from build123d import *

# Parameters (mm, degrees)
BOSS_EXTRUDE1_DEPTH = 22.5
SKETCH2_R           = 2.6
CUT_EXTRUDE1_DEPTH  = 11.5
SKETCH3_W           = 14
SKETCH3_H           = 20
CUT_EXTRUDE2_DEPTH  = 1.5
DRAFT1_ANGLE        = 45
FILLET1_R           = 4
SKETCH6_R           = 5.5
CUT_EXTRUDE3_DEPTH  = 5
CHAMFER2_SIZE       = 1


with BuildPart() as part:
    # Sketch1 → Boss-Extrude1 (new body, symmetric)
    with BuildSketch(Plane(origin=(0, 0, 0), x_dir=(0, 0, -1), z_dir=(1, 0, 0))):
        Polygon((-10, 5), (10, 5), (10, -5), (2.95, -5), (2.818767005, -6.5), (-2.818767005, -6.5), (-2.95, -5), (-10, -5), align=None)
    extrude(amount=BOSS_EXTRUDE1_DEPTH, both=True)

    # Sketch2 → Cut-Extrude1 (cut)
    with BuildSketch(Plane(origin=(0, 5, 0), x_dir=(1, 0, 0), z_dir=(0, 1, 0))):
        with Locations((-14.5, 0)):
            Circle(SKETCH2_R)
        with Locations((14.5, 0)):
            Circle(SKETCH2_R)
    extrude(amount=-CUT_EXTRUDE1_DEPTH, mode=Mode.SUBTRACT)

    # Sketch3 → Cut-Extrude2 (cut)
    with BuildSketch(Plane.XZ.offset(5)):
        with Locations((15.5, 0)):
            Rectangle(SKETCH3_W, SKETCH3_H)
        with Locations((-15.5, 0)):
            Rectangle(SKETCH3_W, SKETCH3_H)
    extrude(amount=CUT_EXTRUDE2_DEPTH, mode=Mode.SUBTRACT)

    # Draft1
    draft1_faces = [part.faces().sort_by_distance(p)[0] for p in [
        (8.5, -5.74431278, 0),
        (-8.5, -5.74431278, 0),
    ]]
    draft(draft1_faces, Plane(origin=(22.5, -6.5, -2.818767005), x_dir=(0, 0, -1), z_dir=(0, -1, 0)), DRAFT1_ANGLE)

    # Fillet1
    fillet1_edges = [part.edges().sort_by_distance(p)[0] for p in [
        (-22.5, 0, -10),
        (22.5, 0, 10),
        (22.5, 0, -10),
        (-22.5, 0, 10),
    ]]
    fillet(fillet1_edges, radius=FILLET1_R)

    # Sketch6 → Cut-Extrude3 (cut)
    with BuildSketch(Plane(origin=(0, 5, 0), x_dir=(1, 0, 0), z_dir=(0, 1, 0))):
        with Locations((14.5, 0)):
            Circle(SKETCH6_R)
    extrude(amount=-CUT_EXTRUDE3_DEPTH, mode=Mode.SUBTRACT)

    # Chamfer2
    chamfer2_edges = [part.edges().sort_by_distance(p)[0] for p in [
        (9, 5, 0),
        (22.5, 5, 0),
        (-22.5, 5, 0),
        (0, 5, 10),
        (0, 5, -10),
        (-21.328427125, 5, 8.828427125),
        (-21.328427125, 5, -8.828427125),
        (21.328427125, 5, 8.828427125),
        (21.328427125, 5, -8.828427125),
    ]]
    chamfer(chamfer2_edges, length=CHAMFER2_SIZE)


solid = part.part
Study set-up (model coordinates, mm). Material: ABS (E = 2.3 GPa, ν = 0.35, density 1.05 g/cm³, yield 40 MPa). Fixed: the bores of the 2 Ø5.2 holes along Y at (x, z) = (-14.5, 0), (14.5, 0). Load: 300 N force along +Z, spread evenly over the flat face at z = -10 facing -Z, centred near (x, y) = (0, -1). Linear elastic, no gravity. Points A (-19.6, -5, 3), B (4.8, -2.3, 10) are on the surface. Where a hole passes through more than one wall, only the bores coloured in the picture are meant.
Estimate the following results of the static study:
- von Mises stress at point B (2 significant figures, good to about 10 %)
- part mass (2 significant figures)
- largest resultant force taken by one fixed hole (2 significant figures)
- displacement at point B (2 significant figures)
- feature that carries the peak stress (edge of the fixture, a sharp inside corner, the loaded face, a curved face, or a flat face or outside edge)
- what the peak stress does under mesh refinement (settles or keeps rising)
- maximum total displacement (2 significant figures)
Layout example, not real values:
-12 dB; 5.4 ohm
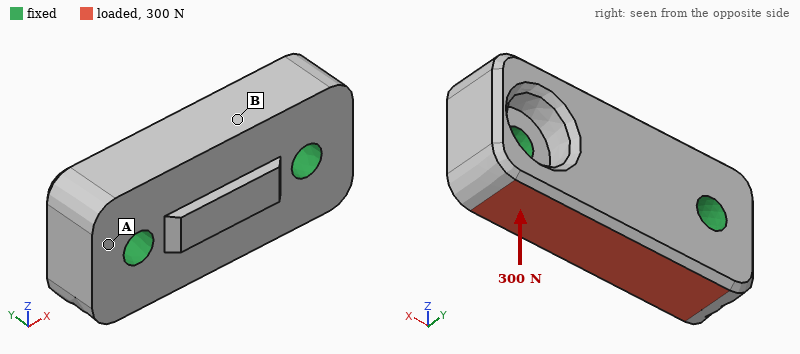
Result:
0.96 MPa; 8.6 g; 160 N; 7.9 µm; edge of the fixture; keeps rising; 16 µm
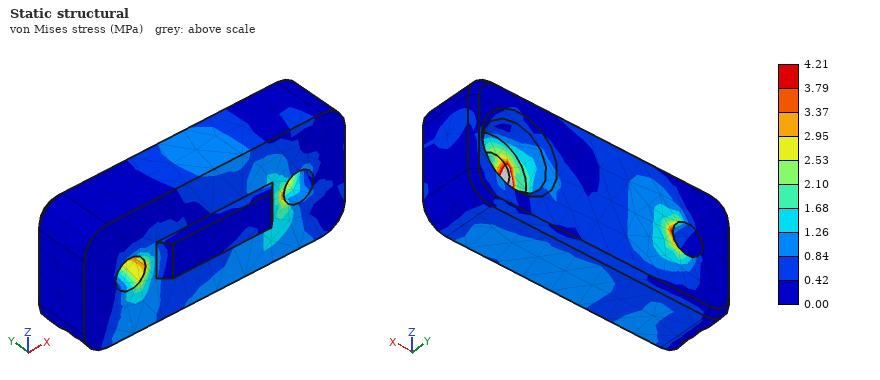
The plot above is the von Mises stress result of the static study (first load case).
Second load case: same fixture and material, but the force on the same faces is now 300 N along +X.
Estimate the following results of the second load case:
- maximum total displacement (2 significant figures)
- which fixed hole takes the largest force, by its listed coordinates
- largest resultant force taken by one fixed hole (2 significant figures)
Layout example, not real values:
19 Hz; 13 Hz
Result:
17 µm; (-14.5, 0); 200 N
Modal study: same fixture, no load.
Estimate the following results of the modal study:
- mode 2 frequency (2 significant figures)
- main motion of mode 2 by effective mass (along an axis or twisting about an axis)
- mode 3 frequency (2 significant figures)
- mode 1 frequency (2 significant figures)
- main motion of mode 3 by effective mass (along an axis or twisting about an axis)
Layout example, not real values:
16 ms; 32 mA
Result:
9200 Hz; along Y; 11 kHz; 7600 Hz; along Z
